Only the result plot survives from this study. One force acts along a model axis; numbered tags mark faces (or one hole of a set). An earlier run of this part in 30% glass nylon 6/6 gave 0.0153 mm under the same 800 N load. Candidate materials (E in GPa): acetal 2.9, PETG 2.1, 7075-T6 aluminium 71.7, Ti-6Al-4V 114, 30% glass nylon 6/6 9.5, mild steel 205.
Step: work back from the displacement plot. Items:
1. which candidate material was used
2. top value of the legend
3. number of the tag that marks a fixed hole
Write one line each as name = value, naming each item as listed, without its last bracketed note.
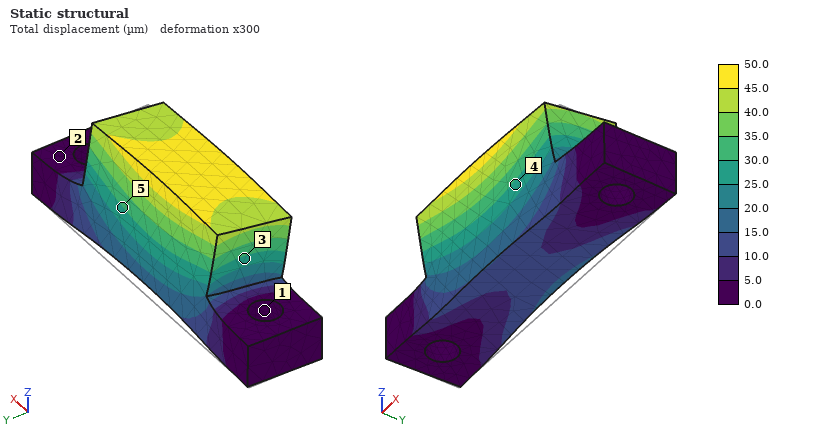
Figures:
which candidate material was used = acetal
top value of the legend = 50.0 µm
number of the tag that marks a fixed hole = 1
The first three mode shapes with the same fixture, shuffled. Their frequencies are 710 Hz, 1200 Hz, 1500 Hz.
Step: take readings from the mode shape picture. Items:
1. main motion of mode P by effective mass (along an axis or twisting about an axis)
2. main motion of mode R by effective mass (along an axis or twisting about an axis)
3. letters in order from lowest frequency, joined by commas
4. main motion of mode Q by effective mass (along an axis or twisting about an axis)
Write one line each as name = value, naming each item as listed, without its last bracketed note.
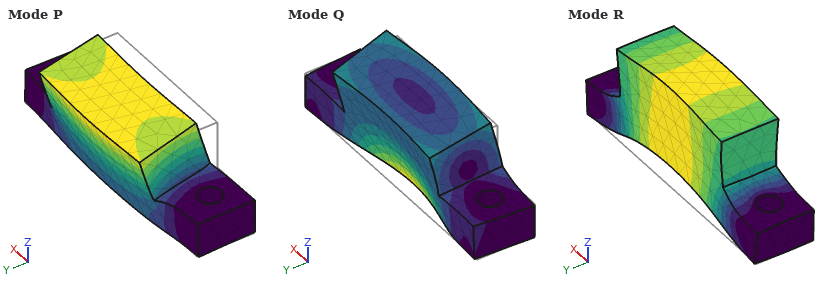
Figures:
main motion of mode P by effective mass = along Y
main motion of mode R by effective mass = along Z
letters in order from lowest frequency, joined by commas = P, R, Q
main motion of mode Q by effective mass = along Y
